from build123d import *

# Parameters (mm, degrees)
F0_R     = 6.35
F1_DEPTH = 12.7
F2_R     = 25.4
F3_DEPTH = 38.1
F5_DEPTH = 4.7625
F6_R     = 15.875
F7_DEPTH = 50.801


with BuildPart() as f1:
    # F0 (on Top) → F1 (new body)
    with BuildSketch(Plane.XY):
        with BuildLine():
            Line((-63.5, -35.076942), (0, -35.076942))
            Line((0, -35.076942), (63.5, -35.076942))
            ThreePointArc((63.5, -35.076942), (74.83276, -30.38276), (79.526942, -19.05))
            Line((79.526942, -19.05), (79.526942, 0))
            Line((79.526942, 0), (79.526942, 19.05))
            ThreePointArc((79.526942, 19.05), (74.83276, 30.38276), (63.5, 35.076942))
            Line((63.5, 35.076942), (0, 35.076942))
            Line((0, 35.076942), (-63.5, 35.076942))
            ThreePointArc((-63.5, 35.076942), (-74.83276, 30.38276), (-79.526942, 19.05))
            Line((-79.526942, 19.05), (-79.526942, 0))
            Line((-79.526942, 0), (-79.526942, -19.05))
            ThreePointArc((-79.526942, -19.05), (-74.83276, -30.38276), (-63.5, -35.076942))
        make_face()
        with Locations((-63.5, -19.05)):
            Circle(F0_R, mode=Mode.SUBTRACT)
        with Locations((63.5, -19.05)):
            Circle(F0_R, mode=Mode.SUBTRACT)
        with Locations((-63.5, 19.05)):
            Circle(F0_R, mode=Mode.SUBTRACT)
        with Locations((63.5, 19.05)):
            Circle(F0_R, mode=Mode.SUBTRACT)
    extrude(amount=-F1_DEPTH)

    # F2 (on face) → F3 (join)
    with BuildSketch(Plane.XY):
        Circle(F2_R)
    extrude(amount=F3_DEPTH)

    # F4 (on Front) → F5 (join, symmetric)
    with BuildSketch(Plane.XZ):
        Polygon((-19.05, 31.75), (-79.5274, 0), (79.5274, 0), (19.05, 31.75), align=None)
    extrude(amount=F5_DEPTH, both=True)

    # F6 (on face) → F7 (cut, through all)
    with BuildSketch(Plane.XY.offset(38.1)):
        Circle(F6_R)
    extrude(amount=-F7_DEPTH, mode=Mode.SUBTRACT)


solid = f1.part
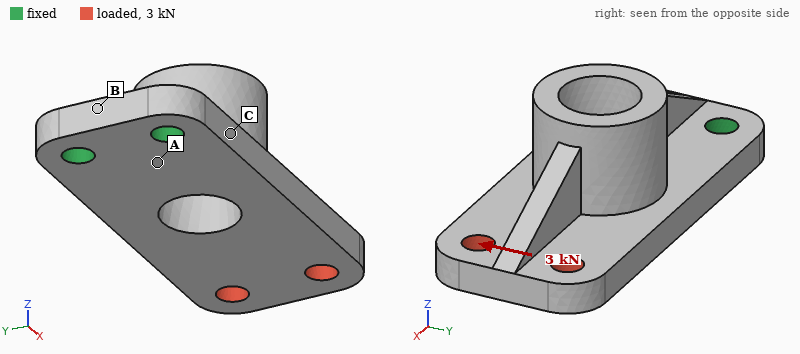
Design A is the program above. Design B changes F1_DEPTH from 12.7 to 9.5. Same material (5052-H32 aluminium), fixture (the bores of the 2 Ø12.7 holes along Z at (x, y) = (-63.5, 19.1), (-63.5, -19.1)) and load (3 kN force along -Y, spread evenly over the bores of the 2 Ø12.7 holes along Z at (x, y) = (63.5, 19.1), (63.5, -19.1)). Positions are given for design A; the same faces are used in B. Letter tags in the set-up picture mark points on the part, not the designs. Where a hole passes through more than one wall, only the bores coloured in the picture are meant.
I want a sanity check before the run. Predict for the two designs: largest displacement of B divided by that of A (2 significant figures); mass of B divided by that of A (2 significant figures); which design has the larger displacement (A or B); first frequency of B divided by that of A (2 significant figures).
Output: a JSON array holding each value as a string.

["1.3", "0.83", "B", "0.84"]
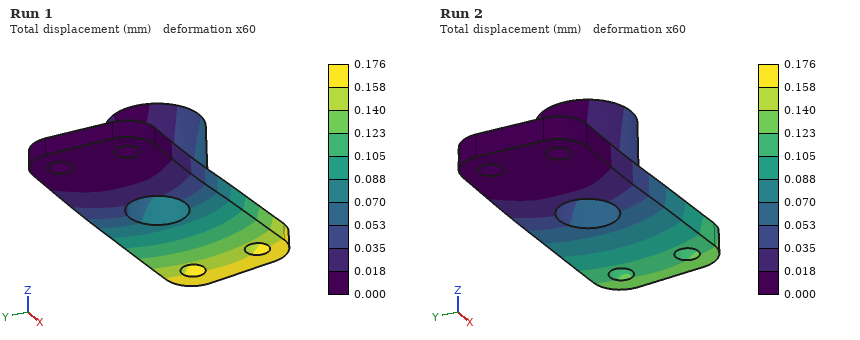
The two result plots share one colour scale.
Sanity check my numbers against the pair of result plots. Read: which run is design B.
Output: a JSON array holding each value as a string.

["Run 1"]
